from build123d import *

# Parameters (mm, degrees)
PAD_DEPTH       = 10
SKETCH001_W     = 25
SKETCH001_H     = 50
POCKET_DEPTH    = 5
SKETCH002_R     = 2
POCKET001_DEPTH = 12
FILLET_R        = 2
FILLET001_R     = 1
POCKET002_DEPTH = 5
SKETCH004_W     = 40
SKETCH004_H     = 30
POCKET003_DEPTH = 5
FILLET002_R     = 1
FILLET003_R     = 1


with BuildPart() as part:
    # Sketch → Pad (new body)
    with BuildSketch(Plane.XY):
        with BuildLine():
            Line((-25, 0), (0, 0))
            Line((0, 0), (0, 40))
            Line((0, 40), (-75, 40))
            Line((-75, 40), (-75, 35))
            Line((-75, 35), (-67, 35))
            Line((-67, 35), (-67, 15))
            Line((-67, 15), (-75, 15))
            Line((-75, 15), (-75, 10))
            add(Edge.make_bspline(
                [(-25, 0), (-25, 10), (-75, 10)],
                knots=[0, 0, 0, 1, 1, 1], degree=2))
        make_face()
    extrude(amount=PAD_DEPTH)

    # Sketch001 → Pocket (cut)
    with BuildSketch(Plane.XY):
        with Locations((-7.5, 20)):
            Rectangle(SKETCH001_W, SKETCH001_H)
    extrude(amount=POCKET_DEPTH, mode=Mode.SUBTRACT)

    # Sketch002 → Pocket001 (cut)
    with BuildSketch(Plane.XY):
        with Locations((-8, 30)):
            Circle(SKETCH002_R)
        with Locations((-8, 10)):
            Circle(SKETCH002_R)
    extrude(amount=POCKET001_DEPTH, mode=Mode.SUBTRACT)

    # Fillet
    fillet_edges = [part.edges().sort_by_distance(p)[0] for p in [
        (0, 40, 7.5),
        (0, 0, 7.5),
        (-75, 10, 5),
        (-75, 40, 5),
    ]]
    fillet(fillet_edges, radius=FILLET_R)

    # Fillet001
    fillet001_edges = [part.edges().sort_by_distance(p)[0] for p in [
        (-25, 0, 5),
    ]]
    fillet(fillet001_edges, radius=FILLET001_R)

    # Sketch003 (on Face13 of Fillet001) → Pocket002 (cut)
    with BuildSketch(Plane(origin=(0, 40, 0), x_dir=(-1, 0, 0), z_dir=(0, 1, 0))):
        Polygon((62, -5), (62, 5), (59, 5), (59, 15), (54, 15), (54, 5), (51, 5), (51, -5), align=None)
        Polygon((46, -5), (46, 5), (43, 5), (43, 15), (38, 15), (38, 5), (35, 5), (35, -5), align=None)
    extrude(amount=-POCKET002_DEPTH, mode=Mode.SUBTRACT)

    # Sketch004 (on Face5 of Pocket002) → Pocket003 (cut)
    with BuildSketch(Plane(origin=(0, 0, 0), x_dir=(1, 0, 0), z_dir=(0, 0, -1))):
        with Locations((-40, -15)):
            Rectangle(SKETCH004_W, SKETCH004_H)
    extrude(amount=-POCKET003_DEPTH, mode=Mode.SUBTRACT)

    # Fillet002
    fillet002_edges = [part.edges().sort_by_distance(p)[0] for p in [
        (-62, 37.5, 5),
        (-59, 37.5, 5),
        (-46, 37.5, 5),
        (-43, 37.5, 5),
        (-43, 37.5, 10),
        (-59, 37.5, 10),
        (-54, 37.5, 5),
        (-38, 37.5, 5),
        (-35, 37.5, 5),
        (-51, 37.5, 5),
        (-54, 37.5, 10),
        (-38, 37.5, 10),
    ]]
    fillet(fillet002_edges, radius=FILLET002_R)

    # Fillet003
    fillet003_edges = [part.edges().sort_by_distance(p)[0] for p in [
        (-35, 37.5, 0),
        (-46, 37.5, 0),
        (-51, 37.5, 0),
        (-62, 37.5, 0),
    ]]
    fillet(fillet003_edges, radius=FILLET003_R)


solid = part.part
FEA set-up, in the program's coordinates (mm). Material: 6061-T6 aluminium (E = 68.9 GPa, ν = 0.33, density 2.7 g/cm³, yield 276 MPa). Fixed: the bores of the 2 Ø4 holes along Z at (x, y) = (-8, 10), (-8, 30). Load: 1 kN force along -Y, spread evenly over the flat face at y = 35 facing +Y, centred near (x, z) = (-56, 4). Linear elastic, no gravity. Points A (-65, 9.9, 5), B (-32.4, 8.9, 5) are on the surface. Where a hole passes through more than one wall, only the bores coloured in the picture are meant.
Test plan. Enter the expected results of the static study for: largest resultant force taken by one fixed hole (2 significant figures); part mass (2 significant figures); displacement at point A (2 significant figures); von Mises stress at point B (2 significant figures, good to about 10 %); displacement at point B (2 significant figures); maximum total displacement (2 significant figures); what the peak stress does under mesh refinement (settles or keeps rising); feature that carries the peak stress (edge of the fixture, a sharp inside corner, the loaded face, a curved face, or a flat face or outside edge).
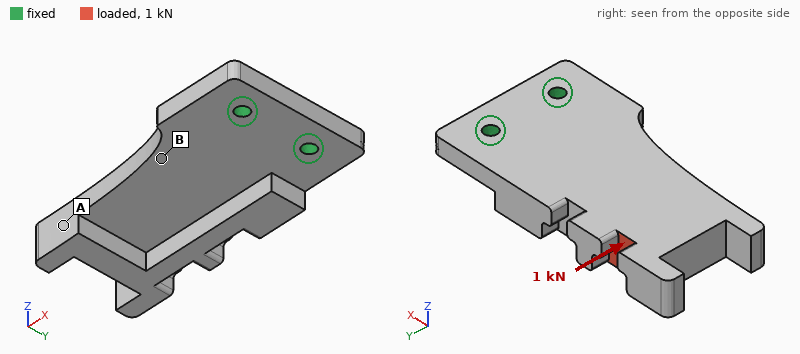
2.2 kN
39 g
0.070 mm
36 MPa
0.024 mm
0.13 mm
keeps rising
edge of the fixture
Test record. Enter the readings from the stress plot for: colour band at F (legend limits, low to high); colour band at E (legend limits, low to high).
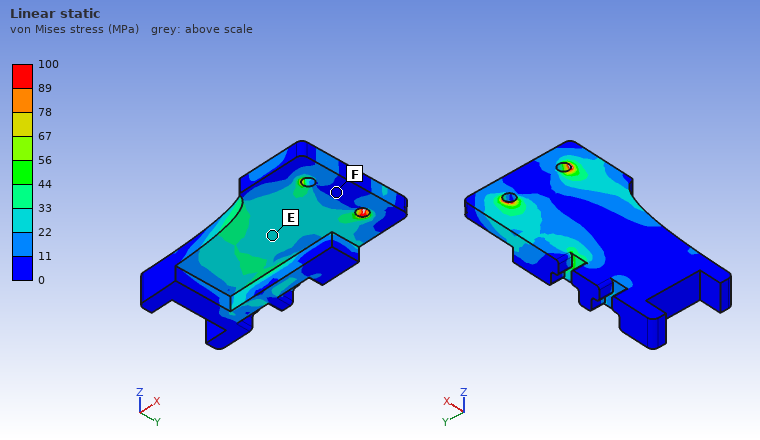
0 to 11 MPa
22 to 33 MPa
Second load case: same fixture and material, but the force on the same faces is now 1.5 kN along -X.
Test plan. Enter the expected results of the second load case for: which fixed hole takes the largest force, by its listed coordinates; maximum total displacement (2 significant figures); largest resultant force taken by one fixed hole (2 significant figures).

(-8, 30)
0.25 mm
1.8 kN
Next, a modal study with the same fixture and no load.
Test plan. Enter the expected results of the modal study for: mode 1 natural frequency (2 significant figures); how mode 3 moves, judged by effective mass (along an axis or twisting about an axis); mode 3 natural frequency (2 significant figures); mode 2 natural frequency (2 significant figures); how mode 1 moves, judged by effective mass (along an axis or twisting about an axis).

1000 Hz
along Y
5000 Hz
3900 Hz
along Z
